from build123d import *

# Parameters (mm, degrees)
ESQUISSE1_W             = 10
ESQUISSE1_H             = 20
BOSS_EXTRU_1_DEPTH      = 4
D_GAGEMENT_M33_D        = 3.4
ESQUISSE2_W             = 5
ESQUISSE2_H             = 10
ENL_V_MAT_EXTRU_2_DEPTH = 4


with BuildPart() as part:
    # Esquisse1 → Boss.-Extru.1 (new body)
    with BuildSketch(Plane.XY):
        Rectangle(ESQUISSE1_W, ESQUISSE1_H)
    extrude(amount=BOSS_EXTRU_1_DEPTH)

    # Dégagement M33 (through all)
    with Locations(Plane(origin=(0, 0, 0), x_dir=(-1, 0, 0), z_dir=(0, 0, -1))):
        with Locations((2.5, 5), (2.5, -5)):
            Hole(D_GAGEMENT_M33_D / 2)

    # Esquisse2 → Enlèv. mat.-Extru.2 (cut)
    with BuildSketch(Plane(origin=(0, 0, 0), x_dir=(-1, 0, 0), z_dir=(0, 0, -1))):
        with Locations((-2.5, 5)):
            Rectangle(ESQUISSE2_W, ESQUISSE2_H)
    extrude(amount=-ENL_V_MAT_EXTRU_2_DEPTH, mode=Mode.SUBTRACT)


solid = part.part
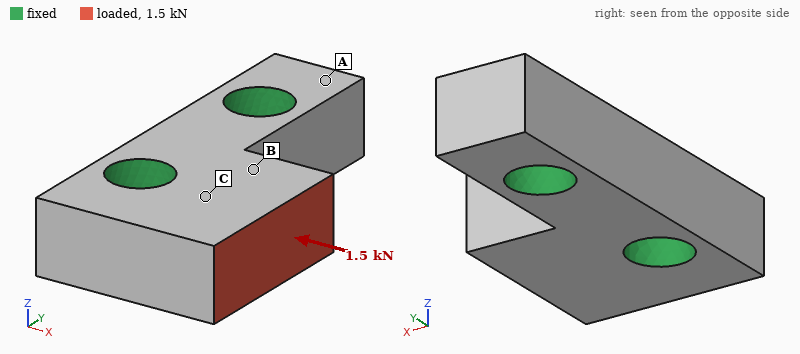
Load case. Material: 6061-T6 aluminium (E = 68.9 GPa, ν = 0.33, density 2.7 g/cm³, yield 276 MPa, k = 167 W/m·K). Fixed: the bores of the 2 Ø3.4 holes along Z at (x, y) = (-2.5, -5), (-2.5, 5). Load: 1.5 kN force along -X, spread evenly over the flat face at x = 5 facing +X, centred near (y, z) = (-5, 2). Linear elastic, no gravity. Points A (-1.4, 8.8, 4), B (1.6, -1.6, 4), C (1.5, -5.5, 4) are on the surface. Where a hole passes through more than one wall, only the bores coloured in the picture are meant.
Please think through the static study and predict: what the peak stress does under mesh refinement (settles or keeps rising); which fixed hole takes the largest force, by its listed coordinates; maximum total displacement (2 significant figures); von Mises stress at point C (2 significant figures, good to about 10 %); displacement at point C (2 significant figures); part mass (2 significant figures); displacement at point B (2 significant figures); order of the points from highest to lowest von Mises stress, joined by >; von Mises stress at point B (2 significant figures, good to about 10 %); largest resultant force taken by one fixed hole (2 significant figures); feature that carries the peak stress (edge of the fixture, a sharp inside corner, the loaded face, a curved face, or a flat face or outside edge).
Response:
keeps rising
(-2.5, -5)
6.3 µm
50 MPa
2.2 µm
1.4 g
2.1 µm
C > B > A
32 MPa
1.4 kN
edge of the fixture
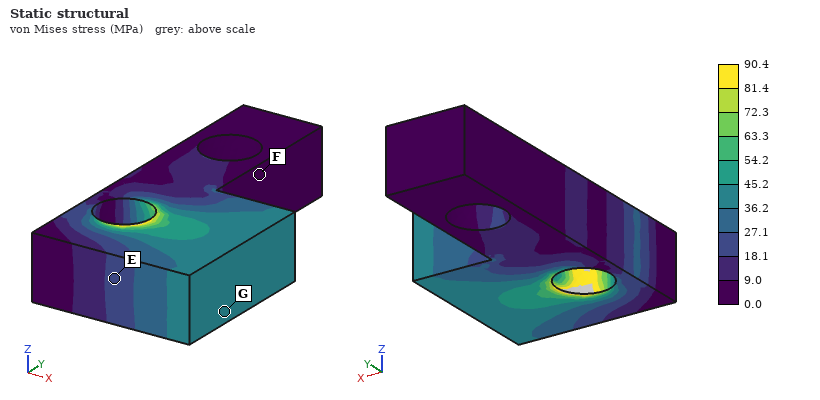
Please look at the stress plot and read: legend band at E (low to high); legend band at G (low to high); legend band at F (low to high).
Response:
18.1 to 27.1 MPa
36.2 to 45.2 MPa
0.0 to 9.0 MPa
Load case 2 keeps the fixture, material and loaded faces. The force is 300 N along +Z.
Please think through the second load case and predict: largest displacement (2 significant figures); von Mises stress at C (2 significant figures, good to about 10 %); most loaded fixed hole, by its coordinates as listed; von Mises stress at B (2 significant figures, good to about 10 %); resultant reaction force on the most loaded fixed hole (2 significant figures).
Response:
12 µm
42 MPa
(-2.5, -5)
34 MPa
300 N
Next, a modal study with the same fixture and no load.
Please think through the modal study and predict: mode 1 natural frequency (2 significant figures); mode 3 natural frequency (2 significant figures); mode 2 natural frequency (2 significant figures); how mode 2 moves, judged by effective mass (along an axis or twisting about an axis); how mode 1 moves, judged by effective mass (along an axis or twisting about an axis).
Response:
57 kHz
77 kHz
70 kHz
along Y
along Z
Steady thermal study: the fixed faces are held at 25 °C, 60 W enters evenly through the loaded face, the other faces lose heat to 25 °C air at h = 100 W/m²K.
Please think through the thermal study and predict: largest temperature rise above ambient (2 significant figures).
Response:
62 K
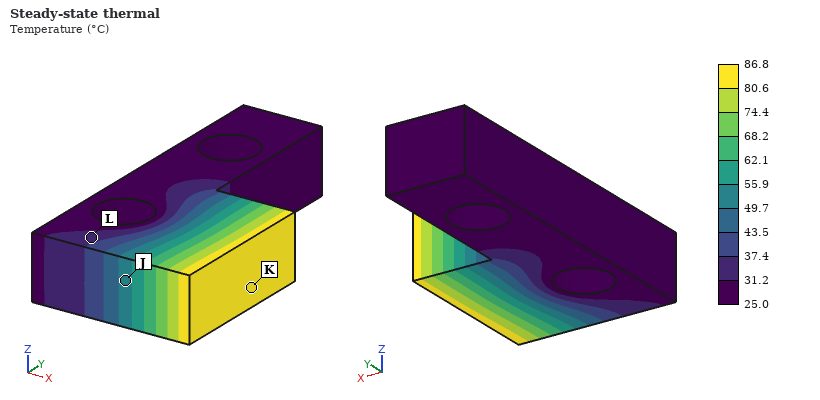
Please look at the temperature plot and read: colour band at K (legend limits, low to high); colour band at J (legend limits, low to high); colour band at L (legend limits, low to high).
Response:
80.6 to 86.8 °C
49.7 to 55.9 °C
31.2 to 37.4 °C
